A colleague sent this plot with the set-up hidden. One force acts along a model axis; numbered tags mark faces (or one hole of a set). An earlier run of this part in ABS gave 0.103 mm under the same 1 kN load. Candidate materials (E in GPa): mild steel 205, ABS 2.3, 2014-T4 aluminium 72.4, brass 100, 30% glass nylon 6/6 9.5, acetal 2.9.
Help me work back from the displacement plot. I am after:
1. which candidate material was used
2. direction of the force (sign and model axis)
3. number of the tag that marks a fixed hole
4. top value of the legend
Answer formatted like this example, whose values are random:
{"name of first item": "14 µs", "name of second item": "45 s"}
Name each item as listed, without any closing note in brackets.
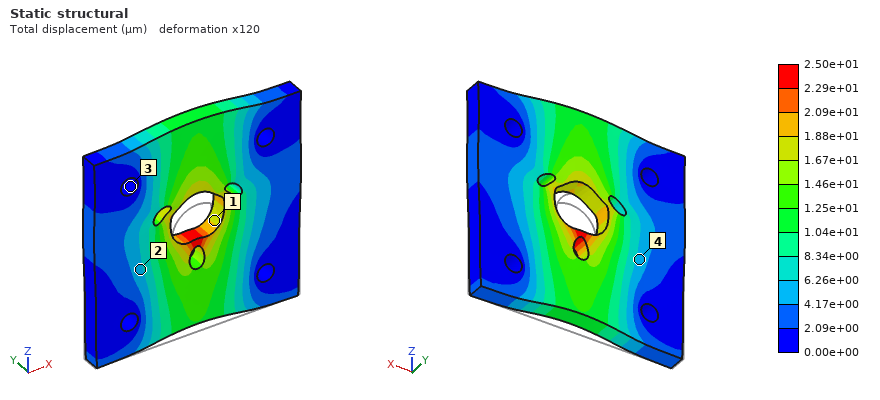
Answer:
{"which candidate material was used": "30% glass nylon 6/6", "direction of the force": "+Z", "number of the tag that marks a fixed hole": "3", "top value of the legend": "2.50e+01 µm"}
